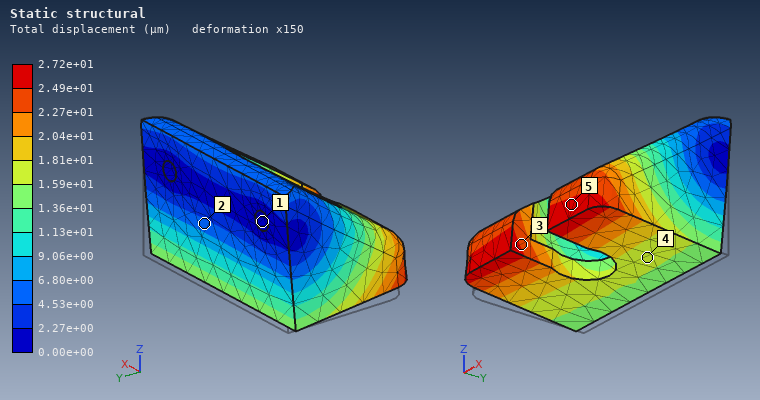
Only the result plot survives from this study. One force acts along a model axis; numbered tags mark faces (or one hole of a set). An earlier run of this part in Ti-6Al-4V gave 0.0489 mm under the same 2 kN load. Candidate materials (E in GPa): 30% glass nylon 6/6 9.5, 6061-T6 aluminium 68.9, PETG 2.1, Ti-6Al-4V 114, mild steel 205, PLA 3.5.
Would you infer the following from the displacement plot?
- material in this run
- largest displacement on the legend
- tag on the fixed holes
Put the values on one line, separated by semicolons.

mild steel; 2.72e+01 µm; 1
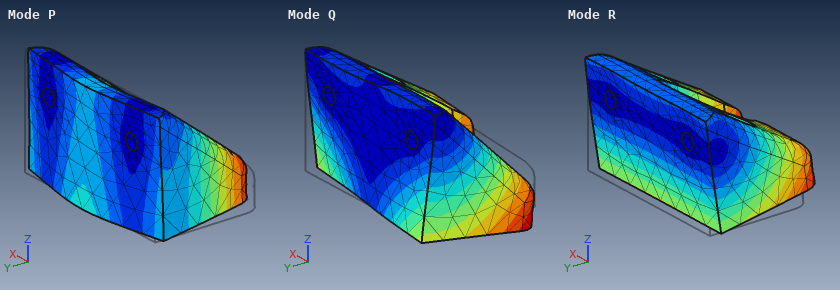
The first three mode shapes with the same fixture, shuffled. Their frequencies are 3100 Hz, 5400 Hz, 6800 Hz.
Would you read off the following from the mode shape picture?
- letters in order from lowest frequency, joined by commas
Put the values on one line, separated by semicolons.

R, Q, P
